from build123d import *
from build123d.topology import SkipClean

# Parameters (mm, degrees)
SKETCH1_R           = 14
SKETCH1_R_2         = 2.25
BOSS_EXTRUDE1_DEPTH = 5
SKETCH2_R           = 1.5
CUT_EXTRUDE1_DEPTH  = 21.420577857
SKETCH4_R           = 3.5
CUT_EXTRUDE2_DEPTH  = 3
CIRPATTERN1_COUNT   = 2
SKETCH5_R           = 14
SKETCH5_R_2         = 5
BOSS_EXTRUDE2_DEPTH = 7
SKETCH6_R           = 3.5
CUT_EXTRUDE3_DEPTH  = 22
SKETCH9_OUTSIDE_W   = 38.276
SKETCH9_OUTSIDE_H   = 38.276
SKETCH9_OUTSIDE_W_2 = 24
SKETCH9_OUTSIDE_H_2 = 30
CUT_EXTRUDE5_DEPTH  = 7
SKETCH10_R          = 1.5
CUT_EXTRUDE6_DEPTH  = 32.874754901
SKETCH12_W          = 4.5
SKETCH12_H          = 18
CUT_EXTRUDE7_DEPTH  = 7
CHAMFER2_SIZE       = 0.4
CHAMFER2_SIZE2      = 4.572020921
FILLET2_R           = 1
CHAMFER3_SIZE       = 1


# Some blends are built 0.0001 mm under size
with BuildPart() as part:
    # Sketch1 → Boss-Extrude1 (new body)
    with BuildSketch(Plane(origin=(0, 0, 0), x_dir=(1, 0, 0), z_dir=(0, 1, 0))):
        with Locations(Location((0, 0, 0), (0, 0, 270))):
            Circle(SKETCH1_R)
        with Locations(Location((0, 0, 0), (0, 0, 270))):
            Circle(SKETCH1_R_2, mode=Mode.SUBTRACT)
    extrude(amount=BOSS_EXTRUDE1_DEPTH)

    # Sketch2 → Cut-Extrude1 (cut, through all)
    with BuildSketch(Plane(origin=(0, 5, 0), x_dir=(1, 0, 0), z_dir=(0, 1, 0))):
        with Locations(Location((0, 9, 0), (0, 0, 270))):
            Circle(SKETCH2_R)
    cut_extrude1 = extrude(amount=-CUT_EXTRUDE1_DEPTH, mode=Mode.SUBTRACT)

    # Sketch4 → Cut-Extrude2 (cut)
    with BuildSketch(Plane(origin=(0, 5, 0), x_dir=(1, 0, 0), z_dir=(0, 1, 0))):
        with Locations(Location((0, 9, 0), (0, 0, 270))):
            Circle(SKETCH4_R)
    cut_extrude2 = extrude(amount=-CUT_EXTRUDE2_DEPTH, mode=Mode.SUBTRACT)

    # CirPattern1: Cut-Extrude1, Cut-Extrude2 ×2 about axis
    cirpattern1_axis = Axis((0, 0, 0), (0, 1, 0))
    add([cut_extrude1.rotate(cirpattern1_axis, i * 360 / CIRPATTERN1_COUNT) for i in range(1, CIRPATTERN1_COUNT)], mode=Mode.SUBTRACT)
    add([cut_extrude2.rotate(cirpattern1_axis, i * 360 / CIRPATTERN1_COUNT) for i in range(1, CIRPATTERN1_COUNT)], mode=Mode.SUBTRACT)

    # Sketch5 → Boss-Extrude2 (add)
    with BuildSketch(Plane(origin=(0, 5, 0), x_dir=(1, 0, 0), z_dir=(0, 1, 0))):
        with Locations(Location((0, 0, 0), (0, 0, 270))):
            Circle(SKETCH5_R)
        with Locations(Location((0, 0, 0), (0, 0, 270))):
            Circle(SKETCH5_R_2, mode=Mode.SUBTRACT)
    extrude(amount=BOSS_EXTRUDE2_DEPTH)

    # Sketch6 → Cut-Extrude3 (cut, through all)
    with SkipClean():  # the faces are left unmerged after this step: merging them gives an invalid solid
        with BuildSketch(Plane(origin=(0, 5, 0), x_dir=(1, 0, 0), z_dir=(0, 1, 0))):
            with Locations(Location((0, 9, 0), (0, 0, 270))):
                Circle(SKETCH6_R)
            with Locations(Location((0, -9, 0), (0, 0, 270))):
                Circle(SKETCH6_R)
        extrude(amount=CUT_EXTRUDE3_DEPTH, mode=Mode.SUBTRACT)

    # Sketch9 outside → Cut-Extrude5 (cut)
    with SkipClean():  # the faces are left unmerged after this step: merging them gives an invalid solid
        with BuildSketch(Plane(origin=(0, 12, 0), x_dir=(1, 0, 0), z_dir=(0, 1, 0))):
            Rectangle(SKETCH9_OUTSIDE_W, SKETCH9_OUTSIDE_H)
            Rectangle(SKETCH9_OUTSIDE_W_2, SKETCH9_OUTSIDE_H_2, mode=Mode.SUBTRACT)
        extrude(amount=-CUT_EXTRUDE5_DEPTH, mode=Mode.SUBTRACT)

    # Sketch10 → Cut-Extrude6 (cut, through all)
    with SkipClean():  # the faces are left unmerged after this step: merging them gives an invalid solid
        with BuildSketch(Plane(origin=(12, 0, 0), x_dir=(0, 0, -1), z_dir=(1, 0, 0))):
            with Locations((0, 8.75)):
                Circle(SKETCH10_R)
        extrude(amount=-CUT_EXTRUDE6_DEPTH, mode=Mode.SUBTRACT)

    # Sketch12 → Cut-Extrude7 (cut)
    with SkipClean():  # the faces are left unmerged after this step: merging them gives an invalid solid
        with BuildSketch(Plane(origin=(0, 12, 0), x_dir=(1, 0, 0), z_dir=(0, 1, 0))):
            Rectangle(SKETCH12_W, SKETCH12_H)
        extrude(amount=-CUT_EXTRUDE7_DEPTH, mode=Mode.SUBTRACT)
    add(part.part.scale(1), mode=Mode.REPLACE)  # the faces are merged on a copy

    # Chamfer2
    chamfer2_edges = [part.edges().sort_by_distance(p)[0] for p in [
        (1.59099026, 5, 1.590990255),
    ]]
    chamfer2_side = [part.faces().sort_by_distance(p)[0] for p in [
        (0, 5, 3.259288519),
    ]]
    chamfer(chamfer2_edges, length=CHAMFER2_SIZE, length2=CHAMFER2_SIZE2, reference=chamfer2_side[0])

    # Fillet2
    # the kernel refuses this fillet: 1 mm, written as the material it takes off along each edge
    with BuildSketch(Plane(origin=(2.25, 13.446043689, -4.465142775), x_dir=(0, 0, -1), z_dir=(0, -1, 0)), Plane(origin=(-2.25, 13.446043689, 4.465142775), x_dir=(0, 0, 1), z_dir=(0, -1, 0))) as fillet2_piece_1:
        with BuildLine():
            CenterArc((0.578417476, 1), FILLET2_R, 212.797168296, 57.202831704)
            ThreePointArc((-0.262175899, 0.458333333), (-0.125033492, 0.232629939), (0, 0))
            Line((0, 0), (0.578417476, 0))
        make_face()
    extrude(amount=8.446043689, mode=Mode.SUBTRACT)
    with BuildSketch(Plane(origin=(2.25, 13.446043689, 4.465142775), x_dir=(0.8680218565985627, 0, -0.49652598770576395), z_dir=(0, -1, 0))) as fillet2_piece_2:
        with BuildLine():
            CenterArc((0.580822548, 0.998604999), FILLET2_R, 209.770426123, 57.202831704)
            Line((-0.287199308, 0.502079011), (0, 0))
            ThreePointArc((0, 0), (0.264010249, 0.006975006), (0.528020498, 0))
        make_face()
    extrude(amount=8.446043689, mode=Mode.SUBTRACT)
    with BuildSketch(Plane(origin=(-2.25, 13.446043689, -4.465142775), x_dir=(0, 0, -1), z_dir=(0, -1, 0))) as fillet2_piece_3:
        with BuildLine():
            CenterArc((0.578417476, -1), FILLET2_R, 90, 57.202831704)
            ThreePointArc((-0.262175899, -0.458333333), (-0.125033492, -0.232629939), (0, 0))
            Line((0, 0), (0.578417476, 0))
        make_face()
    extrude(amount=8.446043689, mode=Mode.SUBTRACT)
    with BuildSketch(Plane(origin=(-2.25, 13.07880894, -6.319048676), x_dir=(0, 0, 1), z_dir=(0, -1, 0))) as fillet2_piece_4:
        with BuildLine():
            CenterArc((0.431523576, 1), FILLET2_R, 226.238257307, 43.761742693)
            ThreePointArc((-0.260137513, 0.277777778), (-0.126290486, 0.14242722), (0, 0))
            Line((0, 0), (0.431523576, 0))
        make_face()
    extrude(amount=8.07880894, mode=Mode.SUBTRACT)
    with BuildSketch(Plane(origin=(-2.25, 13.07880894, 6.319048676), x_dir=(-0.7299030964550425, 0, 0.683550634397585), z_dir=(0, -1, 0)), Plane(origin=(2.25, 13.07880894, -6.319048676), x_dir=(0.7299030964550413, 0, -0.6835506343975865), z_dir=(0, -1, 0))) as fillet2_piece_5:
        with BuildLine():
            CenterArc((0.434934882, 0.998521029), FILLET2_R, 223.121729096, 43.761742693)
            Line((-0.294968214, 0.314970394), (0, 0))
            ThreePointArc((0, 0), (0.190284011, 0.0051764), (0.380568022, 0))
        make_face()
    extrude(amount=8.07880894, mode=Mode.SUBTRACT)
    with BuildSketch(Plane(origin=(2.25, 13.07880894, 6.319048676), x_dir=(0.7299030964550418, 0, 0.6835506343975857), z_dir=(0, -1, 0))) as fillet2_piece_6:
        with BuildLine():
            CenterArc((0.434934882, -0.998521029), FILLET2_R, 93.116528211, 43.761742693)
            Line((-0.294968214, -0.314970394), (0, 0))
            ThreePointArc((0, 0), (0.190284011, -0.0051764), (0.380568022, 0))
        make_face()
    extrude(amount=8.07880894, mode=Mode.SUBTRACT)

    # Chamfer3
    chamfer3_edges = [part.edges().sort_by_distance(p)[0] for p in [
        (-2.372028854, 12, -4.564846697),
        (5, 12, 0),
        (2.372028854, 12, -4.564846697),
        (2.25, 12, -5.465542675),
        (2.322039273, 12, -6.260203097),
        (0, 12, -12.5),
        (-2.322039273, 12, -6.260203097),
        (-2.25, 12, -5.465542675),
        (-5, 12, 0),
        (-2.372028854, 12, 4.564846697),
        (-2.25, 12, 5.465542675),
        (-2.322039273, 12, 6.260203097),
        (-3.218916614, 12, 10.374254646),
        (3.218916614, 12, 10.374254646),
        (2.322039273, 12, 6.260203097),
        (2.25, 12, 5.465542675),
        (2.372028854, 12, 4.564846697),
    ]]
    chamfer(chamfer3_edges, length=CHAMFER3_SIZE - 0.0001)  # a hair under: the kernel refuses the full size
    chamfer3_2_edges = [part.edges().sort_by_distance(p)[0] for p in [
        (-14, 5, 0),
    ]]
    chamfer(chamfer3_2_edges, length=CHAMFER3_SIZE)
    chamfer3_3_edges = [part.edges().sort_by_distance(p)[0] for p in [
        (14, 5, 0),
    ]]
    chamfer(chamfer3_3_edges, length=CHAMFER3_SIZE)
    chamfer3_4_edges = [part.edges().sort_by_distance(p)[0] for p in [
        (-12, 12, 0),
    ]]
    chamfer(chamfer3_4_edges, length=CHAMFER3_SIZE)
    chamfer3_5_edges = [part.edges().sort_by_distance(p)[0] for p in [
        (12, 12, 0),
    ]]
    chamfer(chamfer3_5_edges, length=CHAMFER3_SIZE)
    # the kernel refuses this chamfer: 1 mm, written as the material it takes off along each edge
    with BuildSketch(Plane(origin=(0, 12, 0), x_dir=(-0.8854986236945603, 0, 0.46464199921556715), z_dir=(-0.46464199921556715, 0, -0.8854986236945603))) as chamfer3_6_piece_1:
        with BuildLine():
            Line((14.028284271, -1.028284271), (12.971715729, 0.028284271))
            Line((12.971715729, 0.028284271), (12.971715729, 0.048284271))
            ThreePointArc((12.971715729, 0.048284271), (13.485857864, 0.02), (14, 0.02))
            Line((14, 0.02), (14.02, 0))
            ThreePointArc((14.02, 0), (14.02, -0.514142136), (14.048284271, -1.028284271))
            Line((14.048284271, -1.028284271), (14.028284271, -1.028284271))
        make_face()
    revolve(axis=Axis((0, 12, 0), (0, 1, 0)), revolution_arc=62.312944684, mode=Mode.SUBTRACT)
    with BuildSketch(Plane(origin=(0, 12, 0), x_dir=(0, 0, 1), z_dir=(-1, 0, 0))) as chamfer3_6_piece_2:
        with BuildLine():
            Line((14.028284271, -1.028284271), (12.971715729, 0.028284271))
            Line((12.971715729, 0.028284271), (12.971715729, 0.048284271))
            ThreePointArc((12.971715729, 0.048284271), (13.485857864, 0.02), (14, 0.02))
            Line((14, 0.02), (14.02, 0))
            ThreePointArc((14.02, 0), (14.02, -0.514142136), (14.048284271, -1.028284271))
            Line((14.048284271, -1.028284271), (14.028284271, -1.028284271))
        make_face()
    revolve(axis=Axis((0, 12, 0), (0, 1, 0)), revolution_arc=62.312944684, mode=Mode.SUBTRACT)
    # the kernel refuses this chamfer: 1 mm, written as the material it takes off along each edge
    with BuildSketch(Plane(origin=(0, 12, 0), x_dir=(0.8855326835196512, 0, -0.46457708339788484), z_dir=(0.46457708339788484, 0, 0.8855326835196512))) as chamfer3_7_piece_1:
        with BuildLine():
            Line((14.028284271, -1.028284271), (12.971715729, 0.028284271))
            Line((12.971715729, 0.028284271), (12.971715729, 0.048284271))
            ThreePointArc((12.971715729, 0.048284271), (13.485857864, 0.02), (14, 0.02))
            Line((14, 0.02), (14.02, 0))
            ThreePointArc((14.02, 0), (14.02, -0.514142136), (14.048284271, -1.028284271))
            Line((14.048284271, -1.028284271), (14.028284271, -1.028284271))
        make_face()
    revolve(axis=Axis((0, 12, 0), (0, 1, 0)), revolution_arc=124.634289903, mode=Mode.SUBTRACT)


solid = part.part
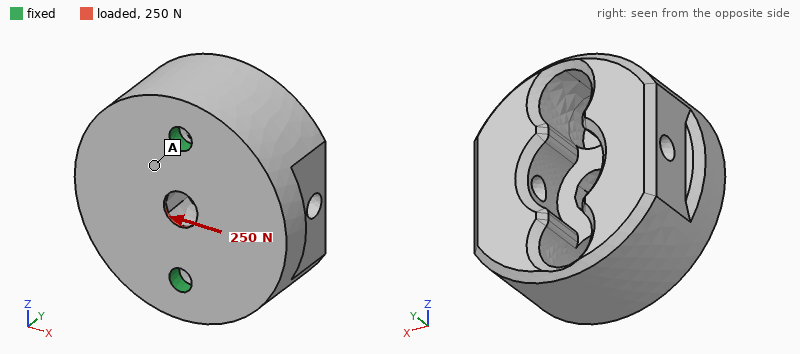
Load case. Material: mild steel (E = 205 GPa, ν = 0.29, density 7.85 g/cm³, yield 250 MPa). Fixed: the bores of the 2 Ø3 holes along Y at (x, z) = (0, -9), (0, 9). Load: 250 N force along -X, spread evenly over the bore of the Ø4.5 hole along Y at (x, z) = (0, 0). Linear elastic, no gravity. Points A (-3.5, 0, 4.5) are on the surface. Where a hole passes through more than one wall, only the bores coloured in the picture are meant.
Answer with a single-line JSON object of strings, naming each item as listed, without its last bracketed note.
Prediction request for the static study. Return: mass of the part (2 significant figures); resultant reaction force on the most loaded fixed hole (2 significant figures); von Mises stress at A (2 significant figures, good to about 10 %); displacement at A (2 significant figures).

{"mass of the part": "43 g", "resultant reaction force on the most loaded fixed hole": "130 N", "von Mises stress at A": "4.8 MPa", "displacement at A": "0.23 µm"}
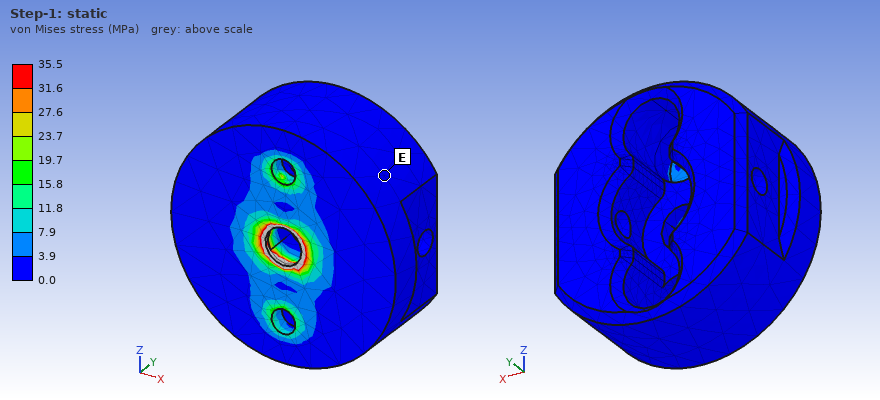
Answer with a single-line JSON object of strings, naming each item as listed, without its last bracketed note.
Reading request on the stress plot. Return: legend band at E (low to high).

{"legend band at E": "0.0 to 3.9 MPa"}
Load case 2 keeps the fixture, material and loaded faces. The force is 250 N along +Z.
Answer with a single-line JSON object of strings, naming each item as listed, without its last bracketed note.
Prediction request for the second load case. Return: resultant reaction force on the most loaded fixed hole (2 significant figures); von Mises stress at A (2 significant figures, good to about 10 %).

{"resultant reaction force on the most loaded fixed hole": "130 N", "von Mises stress at A": "4.2 MPa"}
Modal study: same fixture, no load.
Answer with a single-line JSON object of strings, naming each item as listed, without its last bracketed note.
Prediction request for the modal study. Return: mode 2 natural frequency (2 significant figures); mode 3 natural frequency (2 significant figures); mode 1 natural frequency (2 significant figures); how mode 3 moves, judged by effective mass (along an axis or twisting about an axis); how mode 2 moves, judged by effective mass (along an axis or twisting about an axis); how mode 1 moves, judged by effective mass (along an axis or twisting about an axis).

{"mode 2 natural frequency": "18 kHz", "mode 3 natural frequency": "21 kHz", "mode 1 natural frequency": "5600 Hz", "how mode 3 moves, judged by effective mass": "along Z", "how mode 2 moves, judged by effective mass": "along Y", "how mode 1 moves, judged by effective mass": "along X"}
